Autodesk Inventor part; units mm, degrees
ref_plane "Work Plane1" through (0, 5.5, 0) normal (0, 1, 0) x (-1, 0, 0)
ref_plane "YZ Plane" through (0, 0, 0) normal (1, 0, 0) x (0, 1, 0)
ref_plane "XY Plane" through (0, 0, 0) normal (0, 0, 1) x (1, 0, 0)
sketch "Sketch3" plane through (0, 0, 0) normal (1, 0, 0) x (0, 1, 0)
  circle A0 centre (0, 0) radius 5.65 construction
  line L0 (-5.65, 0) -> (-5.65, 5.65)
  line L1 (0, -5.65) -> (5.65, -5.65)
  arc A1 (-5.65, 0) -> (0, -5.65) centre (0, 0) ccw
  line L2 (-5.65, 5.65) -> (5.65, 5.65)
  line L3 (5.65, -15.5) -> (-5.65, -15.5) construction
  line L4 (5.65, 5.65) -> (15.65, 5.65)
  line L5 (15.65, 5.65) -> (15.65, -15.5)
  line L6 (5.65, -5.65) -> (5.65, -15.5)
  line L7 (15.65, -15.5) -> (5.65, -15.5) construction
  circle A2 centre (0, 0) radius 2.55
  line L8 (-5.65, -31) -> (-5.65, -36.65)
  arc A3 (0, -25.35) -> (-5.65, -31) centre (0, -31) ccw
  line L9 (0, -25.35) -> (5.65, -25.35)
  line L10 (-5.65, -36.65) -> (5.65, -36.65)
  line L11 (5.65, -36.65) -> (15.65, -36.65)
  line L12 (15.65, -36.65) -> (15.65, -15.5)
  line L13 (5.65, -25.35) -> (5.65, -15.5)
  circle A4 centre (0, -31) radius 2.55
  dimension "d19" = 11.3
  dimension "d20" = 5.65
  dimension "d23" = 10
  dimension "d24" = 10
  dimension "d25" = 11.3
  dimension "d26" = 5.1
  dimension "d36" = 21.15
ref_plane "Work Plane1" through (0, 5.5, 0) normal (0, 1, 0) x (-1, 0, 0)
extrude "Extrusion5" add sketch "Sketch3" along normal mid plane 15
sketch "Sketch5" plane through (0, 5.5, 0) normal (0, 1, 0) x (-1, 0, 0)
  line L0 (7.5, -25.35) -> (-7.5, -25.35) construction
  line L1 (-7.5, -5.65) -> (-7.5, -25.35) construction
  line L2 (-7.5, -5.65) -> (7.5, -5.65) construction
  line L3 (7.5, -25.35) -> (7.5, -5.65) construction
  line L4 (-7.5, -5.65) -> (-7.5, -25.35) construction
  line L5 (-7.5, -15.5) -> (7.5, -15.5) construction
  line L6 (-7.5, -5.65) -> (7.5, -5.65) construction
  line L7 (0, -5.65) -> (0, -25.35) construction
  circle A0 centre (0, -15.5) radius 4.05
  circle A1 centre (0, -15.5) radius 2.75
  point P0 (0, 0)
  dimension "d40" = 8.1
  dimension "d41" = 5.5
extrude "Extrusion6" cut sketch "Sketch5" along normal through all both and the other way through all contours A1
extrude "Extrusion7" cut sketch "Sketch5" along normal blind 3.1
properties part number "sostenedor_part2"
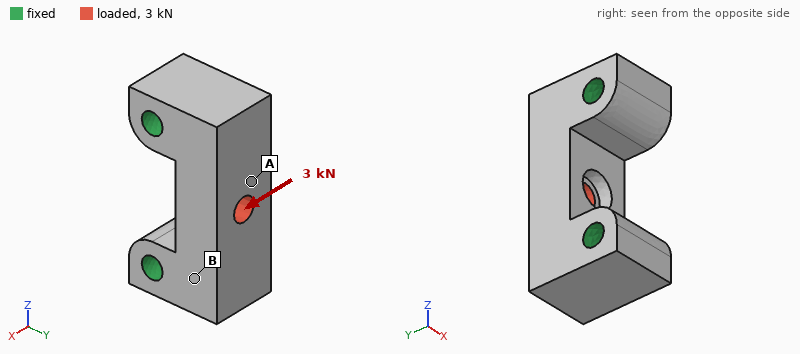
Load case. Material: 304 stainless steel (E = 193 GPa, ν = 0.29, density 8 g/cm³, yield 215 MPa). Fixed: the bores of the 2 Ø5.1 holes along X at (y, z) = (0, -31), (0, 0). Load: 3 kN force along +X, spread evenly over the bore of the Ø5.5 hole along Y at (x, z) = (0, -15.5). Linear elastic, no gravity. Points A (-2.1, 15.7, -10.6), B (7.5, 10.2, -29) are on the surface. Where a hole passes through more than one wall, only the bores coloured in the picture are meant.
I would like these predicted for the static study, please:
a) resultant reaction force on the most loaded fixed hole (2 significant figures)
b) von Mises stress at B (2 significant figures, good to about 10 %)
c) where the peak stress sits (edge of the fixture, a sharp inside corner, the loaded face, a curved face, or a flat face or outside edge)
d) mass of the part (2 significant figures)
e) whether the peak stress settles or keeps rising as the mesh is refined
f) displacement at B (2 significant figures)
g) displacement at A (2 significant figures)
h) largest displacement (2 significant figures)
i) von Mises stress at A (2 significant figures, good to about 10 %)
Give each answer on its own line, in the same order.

1.5 kN
13 MPa
edge of the fixture
72 g
keeps rising
2.7 µm
5.7 µm
6.9 µm
29 MPa
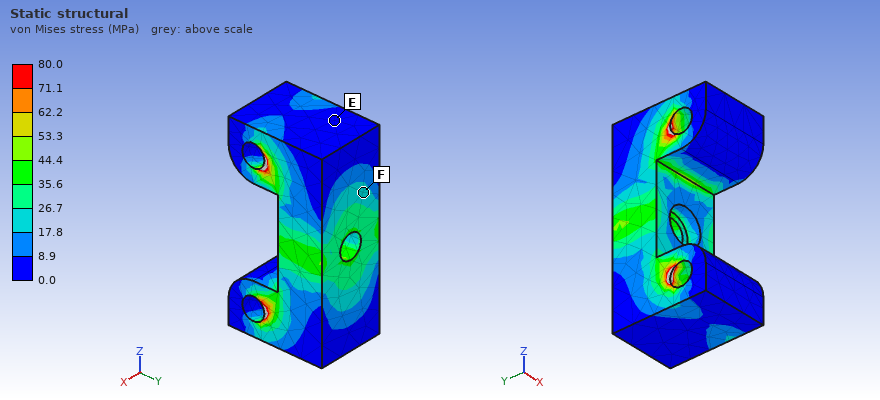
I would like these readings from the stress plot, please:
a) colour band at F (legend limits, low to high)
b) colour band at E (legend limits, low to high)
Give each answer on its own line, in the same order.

17.8 to 26.7 MPa
0.0 to 8.9 MPa
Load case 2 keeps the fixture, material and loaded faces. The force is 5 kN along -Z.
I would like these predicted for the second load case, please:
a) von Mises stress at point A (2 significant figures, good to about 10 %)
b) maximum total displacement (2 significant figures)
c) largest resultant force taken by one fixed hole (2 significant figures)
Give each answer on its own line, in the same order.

30 MPa
4.4 µm
2.7 kN
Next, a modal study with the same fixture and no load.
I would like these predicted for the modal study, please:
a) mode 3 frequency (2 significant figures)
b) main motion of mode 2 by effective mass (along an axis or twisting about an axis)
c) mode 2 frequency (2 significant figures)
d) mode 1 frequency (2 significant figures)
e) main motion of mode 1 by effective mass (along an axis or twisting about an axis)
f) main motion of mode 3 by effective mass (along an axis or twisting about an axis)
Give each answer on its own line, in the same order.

36 kHz
along Z
29 kHz
25 kHz
along X
twisting about Y
